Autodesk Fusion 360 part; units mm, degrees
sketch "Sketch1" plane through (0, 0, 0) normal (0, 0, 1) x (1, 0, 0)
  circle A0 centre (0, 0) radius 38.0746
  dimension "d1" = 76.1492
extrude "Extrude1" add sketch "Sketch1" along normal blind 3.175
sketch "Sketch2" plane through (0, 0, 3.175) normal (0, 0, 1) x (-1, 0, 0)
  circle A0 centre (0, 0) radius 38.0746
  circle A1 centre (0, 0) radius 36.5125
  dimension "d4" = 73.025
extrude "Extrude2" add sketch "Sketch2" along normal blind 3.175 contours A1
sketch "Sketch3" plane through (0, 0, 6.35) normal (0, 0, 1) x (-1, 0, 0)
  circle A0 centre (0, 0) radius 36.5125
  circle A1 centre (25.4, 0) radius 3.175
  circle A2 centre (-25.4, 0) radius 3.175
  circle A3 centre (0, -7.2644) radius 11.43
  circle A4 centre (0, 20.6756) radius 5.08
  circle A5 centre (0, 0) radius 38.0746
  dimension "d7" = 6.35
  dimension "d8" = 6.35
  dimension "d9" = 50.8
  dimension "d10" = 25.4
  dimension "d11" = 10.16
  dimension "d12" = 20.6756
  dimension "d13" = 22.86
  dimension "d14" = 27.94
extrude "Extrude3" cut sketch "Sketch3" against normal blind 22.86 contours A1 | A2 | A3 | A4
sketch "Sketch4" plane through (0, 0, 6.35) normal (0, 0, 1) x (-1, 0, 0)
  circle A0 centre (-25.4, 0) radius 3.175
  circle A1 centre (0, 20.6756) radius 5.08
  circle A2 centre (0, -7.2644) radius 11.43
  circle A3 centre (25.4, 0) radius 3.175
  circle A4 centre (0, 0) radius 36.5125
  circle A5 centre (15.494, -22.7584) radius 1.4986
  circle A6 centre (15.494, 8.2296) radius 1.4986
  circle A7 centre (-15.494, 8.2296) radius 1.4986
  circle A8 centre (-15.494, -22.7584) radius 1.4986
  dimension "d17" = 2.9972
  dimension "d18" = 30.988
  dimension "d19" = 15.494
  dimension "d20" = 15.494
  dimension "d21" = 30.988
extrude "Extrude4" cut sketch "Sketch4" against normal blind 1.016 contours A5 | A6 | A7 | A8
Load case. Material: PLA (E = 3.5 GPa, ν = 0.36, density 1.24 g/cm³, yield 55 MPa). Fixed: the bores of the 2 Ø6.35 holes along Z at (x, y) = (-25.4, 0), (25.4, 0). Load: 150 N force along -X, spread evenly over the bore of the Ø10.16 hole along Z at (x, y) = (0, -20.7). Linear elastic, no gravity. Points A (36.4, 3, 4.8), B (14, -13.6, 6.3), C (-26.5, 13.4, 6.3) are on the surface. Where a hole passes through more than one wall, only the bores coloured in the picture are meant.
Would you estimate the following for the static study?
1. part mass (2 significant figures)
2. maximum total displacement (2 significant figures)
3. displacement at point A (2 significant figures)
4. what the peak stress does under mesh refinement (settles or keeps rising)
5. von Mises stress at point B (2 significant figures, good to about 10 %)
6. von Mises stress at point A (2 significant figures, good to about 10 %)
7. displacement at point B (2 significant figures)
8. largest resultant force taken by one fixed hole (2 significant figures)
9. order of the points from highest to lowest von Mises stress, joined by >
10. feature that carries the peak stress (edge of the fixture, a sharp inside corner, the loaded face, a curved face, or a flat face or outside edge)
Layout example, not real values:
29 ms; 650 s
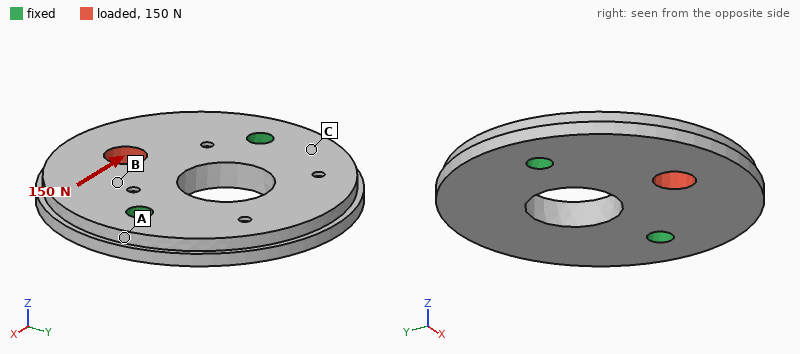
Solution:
30 g; 12 µm; 2.0 µm; keeps rising; 0.68 MPa; 0.41 MPa; 5.7 µm; 92 N; B > A > C; edge of the fixture
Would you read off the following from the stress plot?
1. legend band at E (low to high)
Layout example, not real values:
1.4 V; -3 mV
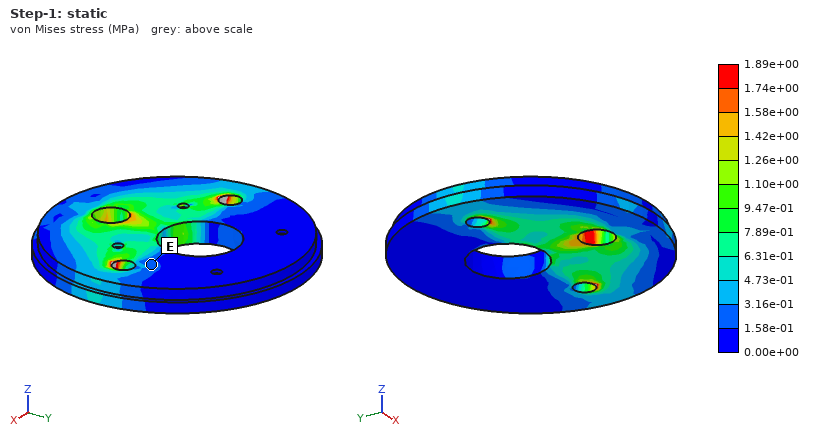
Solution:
1.58e-01 to 3.16e-01 MPa
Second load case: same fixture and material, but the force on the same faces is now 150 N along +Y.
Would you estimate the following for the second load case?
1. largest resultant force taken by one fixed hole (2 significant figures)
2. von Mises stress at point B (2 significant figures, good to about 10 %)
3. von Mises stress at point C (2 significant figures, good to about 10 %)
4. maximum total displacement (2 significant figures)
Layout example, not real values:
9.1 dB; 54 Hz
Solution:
83 N; 0.62 MPa; 0.19 MPa; 9.1 µm
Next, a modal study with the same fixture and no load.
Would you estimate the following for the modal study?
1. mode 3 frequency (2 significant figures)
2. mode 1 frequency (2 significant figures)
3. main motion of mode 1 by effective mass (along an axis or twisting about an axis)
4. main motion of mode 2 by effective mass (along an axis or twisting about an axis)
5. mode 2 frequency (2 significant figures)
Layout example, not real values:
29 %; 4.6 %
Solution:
3000 Hz; 1200 Hz; twisting about X; along Z; 1400 Hz
